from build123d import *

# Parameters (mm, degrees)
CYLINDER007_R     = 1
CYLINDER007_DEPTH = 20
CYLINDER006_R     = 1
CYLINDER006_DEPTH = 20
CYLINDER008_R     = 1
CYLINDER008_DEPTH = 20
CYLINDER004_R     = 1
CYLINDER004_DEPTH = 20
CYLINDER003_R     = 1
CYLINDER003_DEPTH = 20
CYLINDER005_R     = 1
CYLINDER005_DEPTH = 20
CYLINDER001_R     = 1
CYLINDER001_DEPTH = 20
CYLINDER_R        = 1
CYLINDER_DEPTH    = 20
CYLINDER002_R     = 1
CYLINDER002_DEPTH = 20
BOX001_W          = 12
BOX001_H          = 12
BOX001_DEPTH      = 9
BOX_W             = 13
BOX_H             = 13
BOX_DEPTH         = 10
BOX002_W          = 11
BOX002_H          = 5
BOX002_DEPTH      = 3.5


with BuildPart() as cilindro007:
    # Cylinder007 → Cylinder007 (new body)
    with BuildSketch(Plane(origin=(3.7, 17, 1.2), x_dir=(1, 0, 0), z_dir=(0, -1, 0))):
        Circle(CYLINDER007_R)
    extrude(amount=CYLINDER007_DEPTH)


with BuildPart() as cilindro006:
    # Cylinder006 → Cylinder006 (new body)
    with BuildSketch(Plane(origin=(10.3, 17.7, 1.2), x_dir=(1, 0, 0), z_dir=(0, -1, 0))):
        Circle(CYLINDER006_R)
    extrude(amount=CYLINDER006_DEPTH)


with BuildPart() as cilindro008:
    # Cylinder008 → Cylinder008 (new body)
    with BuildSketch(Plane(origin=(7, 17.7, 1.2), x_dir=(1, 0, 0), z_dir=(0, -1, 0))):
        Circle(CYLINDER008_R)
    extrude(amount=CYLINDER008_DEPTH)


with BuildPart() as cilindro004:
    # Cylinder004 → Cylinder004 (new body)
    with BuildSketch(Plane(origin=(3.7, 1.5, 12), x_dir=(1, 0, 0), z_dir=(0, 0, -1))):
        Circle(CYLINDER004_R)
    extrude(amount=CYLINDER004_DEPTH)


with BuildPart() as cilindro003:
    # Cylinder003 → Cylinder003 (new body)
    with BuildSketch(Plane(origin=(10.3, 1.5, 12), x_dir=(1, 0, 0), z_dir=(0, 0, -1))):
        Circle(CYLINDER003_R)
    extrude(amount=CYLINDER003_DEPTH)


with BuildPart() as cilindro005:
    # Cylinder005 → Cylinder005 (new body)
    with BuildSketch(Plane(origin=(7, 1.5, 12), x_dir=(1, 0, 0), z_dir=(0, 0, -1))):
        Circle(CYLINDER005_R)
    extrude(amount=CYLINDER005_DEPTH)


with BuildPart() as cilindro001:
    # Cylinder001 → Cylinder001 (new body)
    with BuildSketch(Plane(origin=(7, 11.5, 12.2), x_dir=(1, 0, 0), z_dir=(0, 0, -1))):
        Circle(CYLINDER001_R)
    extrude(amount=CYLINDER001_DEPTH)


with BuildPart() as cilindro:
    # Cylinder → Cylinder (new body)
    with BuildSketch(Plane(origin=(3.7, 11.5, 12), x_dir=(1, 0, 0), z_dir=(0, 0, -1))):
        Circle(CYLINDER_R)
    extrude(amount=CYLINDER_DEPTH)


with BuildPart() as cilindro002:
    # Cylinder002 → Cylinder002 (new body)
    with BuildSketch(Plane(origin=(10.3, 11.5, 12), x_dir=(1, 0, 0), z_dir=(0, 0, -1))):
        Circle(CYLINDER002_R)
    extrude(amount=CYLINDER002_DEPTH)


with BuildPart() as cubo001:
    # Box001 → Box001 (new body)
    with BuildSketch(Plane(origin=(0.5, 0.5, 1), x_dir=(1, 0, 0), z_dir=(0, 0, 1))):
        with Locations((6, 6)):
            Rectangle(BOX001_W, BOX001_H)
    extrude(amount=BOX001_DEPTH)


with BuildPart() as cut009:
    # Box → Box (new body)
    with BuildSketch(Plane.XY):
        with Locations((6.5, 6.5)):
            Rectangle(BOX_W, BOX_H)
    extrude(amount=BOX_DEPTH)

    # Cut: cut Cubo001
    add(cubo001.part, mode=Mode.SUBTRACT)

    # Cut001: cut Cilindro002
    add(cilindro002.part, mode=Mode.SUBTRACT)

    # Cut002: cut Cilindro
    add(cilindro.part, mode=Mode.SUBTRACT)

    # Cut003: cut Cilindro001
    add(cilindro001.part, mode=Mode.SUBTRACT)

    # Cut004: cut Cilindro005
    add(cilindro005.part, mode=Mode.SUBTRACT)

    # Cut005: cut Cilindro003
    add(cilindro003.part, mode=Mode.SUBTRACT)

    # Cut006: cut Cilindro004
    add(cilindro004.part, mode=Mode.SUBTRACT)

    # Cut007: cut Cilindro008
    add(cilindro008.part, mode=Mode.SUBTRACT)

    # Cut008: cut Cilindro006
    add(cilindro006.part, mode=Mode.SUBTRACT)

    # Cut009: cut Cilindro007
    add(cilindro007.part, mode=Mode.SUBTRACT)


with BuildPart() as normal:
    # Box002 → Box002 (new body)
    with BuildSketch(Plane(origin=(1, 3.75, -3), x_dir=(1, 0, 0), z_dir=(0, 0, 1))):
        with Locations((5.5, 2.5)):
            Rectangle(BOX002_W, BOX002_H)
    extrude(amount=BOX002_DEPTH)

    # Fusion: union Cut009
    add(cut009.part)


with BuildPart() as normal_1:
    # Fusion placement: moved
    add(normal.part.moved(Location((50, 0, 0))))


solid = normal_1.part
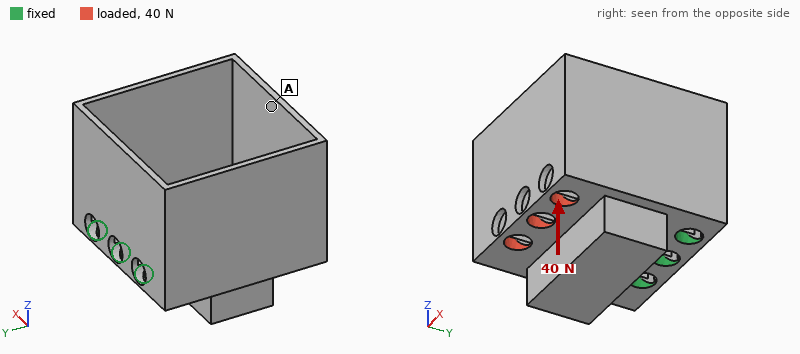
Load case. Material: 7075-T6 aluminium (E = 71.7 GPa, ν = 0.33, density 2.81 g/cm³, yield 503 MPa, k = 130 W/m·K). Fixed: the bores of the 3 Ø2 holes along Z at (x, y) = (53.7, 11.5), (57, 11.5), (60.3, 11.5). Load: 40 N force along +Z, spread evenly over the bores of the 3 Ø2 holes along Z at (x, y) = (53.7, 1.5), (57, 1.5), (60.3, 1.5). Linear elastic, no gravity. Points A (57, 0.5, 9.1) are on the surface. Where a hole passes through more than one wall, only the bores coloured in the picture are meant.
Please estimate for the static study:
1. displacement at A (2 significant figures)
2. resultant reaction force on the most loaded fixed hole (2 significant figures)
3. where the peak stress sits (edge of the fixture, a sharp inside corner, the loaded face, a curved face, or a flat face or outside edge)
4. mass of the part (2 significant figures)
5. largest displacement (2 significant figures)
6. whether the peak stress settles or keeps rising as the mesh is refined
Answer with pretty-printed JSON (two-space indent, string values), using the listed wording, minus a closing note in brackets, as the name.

{
  "displacement at A": "78 µm",
  "resultant reaction force on the most loaded fixed hole": "24 N",
  "where the peak stress sits": "edge of the fixture",
  "mass of the part": "1.4 g",
  "largest displacement": "85 µm",
  "whether the peak stress settles or keeps rising as the mesh is refined": "keeps rising"
}
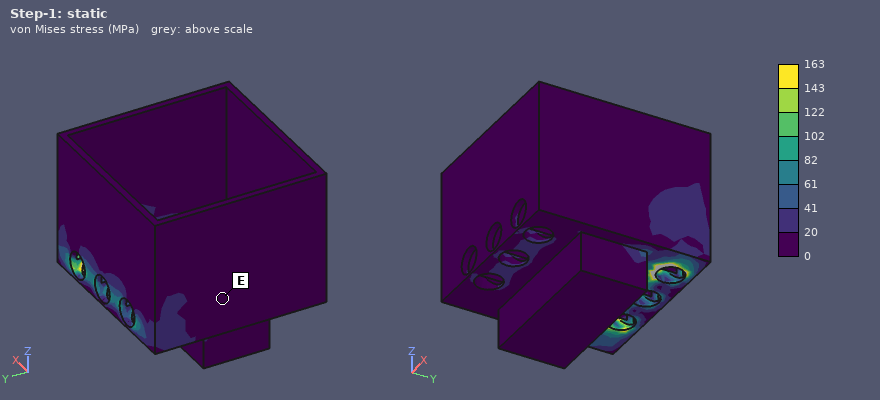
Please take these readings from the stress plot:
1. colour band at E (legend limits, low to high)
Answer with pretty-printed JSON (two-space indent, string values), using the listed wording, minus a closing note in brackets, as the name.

{
  "colour band at E": "0 to 20 MPa"
}
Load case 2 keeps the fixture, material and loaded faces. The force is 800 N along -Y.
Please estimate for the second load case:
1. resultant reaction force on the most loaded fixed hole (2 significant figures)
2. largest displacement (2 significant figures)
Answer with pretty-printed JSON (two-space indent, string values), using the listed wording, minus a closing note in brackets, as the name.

{
  "resultant reaction force on the most loaded fixed hole": "290 N",
  "largest displacement": "23 µm"
}
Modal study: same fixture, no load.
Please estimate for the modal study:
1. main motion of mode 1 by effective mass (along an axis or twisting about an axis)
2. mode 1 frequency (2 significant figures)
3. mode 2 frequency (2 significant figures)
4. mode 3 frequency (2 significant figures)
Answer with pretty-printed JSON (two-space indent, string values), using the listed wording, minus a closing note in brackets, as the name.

{
  "main motion of mode 1 by effective mass": "along Z",
  "mode 1 frequency": "4800 Hz",
  "mode 2 frequency": "8400 Hz",
  "mode 3 frequency": "11 kHz"
}
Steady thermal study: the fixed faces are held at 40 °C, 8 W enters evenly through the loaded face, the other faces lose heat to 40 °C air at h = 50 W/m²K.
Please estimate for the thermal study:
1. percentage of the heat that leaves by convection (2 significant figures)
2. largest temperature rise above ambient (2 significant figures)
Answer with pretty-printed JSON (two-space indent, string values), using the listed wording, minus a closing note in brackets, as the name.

{
  "percentage of the heat that leaves by convection": "14 %",
  "largest temperature rise above ambient": "44 K"
}
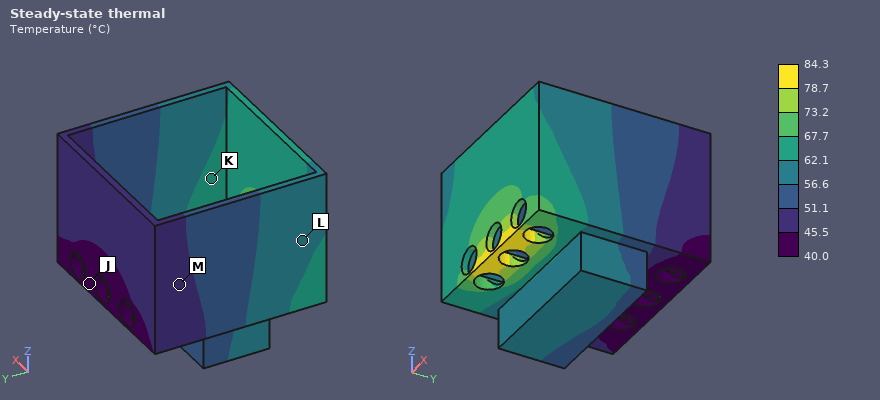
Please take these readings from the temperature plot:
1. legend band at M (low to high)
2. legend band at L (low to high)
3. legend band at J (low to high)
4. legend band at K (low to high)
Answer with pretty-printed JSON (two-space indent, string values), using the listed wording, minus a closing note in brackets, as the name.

{
  "legend band at M": "45.5 to 51.1 °C",
  "legend band at L": "56.6 to 62.1 °C",
  "legend band at J": "40.0 to 45.5 °C",
  "legend band at K": "62.1 to 67.7 °C"
}
